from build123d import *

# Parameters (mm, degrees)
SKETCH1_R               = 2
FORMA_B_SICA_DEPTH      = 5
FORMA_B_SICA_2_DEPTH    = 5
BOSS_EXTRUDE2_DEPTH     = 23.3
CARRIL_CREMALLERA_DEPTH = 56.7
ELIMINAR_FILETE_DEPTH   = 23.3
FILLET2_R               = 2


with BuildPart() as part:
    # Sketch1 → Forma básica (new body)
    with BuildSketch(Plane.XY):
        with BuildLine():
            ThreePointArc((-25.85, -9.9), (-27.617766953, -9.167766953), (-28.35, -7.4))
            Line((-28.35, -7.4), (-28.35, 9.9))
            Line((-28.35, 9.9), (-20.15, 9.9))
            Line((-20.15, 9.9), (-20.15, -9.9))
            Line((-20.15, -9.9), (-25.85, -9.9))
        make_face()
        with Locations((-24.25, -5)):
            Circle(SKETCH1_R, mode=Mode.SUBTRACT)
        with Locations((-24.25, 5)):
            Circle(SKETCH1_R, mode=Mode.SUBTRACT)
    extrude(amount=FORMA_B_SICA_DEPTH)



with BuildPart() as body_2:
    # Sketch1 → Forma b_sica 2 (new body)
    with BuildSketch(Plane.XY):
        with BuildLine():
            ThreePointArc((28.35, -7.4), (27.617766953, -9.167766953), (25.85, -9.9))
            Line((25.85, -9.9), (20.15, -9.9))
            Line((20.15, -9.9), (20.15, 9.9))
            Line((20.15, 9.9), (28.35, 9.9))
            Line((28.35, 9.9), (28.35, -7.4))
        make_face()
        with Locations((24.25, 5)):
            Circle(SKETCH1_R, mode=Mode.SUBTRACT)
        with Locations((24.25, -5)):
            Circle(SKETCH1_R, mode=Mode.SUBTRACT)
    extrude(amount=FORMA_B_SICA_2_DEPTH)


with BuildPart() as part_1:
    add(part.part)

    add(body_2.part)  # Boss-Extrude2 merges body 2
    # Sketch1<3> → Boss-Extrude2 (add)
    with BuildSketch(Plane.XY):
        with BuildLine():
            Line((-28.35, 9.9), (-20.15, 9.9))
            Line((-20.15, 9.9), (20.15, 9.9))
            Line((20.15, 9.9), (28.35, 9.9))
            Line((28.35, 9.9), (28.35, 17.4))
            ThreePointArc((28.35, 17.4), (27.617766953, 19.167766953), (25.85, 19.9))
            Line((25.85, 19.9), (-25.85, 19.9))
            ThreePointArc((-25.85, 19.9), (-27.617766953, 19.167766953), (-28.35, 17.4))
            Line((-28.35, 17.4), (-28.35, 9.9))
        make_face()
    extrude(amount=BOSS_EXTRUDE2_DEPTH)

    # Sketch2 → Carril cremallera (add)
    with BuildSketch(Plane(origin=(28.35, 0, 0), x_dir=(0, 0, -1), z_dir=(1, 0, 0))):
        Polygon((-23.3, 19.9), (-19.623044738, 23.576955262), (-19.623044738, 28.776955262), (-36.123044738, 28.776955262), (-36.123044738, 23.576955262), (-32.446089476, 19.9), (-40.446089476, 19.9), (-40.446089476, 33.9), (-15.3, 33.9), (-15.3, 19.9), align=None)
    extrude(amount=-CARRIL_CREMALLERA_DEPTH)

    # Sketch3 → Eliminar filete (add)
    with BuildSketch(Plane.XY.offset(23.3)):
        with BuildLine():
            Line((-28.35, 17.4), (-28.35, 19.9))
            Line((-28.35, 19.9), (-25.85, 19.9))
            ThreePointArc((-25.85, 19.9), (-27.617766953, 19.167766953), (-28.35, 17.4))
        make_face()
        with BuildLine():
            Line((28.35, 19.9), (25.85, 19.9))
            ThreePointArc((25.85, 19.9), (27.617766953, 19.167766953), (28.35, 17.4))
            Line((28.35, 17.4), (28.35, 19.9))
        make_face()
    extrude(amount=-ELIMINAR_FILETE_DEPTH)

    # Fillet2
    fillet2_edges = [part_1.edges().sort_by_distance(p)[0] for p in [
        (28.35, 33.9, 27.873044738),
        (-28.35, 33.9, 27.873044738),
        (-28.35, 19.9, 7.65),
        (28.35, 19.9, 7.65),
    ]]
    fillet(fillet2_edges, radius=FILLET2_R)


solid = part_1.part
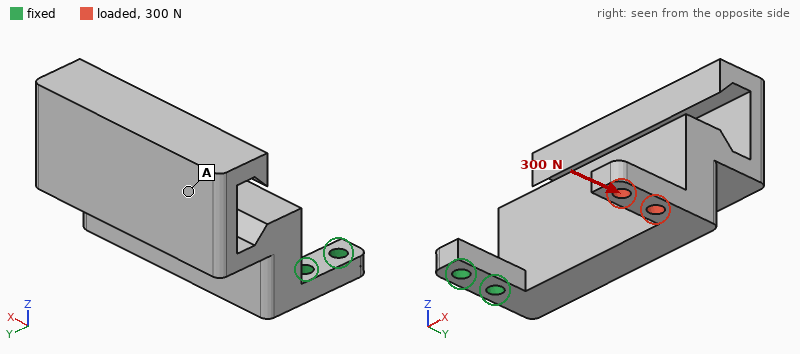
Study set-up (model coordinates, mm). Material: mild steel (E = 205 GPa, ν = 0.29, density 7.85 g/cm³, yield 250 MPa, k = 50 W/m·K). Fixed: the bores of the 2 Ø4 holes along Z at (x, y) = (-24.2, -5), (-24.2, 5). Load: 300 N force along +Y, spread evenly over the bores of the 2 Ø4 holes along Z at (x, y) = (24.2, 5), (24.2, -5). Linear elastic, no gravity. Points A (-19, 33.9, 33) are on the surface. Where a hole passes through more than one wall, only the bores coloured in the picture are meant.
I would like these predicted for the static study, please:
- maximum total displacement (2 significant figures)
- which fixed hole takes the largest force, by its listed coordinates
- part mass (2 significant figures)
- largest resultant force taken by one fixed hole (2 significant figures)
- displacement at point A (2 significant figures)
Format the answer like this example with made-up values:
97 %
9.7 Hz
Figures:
0.18 mm
(-24.2, 5)
210 g
420 N
0.069 mm
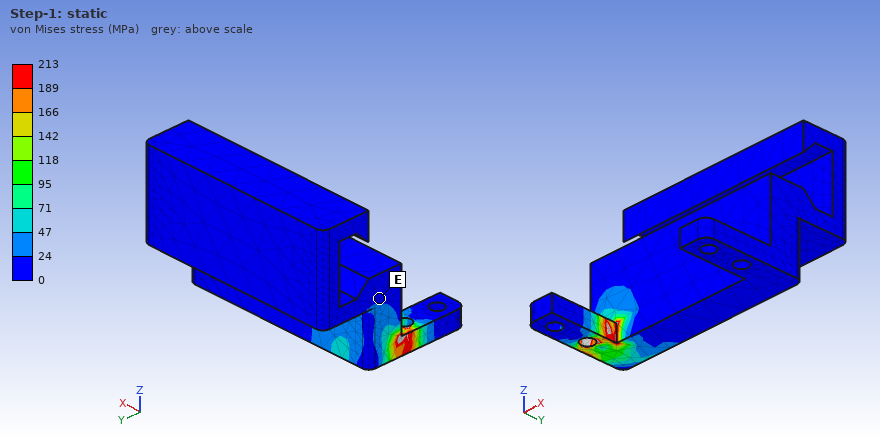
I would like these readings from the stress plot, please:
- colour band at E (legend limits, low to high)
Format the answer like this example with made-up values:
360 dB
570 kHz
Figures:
0 to 24 MPa
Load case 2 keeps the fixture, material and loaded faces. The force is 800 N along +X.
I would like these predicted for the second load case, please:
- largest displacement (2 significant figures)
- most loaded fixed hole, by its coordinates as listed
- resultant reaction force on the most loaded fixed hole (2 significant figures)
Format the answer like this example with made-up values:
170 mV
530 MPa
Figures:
0.13 mm
(-24.2, 5)
700 N
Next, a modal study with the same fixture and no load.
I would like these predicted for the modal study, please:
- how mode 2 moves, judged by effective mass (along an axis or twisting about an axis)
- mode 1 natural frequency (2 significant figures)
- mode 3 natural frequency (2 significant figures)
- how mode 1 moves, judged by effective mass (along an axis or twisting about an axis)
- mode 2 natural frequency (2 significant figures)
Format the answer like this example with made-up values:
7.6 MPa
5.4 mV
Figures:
along Y
540 Hz
1200 Hz
along Z
610 Hz
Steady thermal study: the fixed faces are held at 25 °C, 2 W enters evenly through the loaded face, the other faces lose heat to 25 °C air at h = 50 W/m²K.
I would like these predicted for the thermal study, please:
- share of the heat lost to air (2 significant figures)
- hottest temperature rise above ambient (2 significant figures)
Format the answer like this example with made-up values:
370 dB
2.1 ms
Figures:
77 %
18 K
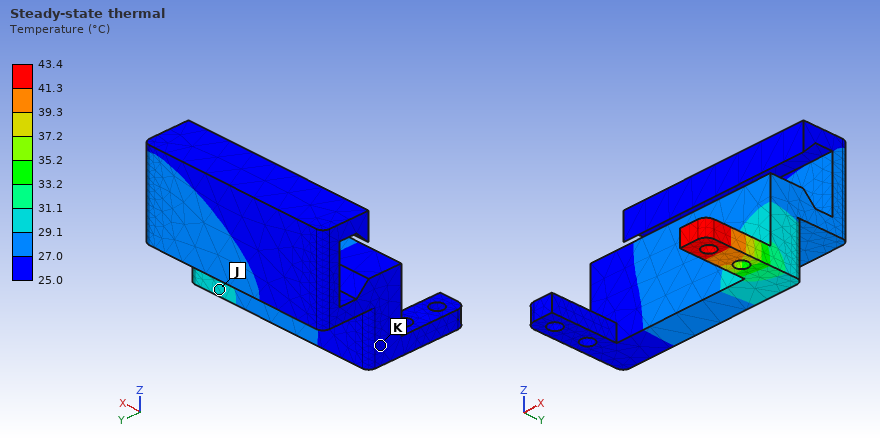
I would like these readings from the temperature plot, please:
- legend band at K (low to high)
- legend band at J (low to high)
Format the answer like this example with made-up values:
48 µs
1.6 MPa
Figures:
25.0 to 27.0 °C
29.1 to 31.1 °C
